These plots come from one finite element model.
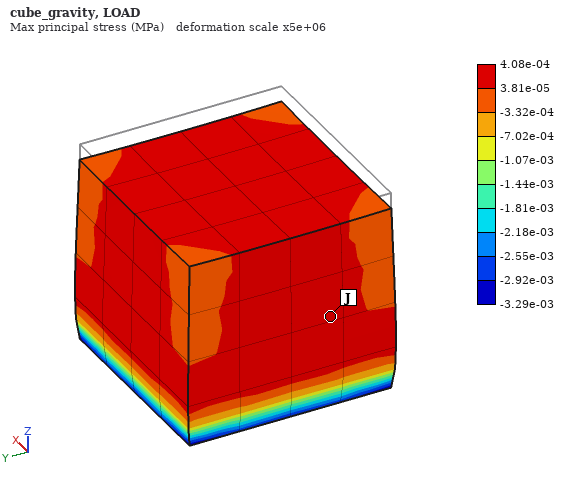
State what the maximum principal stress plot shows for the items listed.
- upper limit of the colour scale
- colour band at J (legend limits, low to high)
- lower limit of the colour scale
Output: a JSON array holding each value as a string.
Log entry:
["4.08e-04 MPa", "3.81e-05 to 4.08e-04 MPa", "-3.29e-03 MPa"]
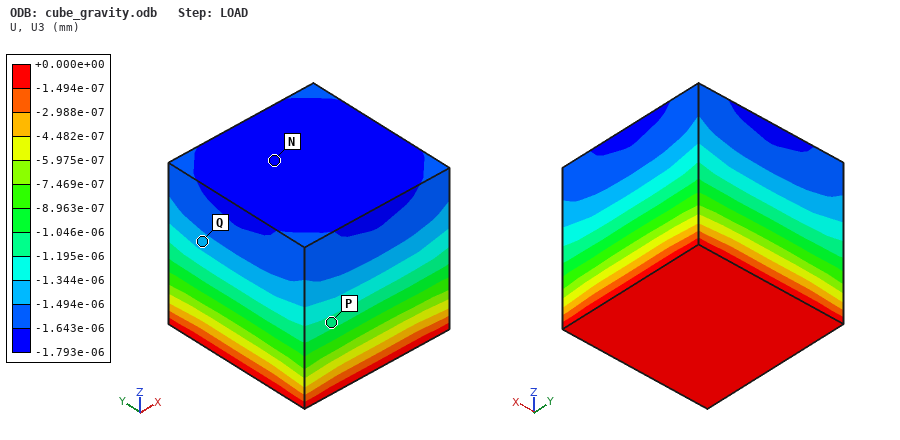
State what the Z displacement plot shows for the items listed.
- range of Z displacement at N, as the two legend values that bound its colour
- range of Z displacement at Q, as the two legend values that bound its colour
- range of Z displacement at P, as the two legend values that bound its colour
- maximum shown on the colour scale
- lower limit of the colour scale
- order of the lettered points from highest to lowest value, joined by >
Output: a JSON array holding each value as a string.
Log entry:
["-1.793e-06 to -1.643e-06 mm", "-1.494e-06 to -1.344e-06 mm", "-1.195e-06 to -1.046e-06 mm", "+0.000e+00 mm", "-1.793e-06 mm", "P > Q > N"]
